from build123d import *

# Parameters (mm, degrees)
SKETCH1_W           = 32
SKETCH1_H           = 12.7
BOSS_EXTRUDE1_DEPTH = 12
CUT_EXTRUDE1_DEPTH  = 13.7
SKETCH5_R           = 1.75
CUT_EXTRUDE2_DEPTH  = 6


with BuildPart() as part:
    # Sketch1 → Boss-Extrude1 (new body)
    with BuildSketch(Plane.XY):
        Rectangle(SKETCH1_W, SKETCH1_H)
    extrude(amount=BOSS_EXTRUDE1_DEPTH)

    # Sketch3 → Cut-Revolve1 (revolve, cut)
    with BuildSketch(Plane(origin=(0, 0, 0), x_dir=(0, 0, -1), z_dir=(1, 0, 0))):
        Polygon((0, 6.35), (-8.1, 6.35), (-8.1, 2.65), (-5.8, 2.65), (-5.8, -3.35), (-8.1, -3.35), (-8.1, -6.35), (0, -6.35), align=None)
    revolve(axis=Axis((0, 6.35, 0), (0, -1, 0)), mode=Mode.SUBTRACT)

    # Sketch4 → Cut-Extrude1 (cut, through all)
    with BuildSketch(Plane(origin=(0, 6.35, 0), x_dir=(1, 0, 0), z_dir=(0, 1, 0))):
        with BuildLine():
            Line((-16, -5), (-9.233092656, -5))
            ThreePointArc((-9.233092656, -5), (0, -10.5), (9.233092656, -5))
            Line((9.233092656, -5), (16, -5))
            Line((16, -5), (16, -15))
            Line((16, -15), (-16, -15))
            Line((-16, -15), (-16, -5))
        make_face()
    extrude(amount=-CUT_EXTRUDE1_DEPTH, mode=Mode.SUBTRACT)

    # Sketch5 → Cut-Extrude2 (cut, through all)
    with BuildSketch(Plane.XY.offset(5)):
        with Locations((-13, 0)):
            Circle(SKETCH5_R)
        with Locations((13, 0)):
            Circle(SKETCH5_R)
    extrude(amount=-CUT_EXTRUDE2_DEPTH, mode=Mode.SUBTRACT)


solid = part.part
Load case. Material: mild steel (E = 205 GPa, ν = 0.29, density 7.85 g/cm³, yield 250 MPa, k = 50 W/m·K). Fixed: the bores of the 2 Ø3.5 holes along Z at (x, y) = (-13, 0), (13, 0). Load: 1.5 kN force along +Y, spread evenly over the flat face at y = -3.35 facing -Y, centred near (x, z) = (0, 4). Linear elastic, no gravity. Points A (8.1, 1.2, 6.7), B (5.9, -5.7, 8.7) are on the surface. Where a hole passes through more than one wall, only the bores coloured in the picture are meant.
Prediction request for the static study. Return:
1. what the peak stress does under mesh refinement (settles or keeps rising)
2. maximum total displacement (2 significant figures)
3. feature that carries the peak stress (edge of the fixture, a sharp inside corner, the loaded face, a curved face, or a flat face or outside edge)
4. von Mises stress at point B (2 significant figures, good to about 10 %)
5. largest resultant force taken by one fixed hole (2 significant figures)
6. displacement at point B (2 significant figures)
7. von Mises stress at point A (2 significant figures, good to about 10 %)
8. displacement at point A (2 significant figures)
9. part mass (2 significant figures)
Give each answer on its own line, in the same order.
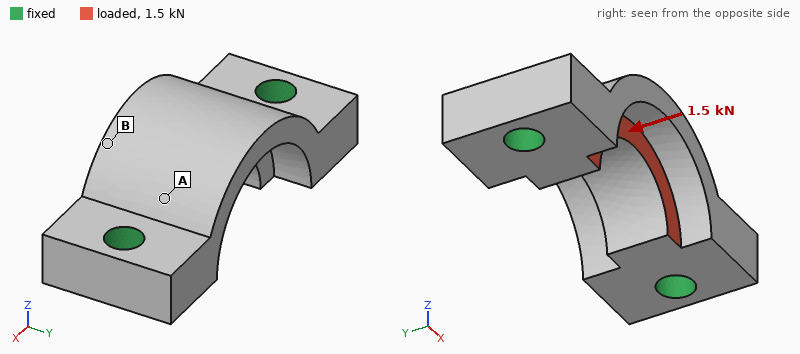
keeps rising
6.9 µm
edge of the fixture
15 MPa
750 N
4.9 µm
40 MPa
3.1 µm
14 g
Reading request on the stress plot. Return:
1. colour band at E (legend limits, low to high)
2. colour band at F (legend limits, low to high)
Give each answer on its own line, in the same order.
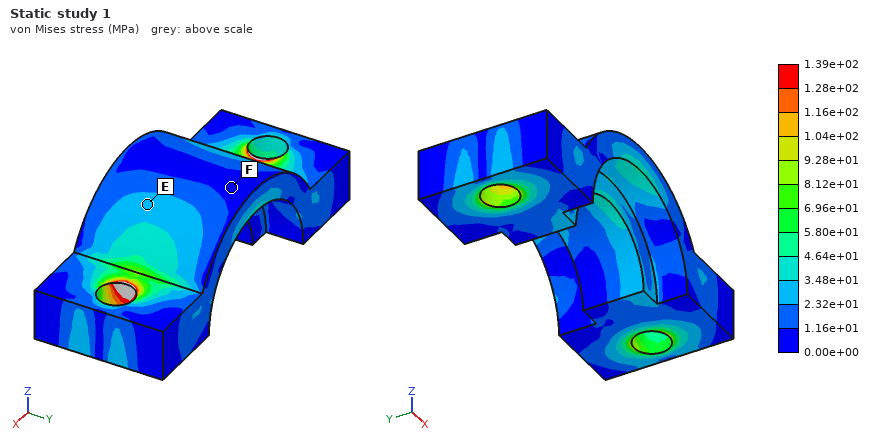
2.32e+01 to 3.48e+01 MPa
0.00e+00 to 1.16e+01 MPa
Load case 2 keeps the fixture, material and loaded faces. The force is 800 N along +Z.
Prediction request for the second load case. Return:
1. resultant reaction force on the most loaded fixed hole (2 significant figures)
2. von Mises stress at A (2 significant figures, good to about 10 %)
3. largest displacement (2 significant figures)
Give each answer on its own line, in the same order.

490 N
17 MPa
3.6 µm
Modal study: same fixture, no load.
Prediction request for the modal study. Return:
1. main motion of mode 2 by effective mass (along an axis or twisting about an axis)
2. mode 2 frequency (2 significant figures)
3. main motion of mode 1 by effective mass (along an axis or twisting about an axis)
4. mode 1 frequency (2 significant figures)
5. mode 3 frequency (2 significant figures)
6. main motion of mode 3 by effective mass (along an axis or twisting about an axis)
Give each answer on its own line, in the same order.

along Z
45 kHz
along Y
26 kHz
56 kHz
along X
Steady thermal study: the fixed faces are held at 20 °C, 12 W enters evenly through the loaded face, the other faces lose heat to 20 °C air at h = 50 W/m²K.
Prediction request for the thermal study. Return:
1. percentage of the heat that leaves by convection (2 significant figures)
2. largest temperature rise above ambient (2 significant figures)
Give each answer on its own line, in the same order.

5.2 %
28 K
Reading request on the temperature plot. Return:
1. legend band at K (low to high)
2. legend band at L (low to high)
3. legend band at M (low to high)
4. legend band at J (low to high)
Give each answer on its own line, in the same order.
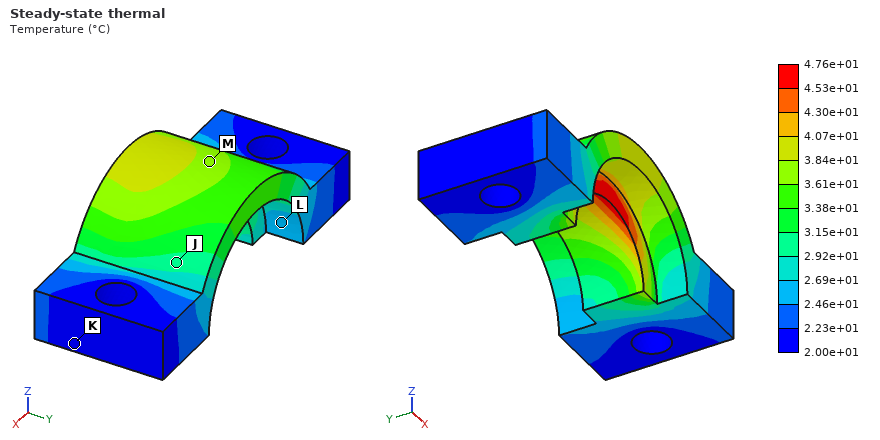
2.00e+01 to 2.23e+01 °C
2.46e+01 to 2.69e+01 °C
3.61e+01 to 3.84e+01 °C
2.92e+01 to 3.15e+01 °C
